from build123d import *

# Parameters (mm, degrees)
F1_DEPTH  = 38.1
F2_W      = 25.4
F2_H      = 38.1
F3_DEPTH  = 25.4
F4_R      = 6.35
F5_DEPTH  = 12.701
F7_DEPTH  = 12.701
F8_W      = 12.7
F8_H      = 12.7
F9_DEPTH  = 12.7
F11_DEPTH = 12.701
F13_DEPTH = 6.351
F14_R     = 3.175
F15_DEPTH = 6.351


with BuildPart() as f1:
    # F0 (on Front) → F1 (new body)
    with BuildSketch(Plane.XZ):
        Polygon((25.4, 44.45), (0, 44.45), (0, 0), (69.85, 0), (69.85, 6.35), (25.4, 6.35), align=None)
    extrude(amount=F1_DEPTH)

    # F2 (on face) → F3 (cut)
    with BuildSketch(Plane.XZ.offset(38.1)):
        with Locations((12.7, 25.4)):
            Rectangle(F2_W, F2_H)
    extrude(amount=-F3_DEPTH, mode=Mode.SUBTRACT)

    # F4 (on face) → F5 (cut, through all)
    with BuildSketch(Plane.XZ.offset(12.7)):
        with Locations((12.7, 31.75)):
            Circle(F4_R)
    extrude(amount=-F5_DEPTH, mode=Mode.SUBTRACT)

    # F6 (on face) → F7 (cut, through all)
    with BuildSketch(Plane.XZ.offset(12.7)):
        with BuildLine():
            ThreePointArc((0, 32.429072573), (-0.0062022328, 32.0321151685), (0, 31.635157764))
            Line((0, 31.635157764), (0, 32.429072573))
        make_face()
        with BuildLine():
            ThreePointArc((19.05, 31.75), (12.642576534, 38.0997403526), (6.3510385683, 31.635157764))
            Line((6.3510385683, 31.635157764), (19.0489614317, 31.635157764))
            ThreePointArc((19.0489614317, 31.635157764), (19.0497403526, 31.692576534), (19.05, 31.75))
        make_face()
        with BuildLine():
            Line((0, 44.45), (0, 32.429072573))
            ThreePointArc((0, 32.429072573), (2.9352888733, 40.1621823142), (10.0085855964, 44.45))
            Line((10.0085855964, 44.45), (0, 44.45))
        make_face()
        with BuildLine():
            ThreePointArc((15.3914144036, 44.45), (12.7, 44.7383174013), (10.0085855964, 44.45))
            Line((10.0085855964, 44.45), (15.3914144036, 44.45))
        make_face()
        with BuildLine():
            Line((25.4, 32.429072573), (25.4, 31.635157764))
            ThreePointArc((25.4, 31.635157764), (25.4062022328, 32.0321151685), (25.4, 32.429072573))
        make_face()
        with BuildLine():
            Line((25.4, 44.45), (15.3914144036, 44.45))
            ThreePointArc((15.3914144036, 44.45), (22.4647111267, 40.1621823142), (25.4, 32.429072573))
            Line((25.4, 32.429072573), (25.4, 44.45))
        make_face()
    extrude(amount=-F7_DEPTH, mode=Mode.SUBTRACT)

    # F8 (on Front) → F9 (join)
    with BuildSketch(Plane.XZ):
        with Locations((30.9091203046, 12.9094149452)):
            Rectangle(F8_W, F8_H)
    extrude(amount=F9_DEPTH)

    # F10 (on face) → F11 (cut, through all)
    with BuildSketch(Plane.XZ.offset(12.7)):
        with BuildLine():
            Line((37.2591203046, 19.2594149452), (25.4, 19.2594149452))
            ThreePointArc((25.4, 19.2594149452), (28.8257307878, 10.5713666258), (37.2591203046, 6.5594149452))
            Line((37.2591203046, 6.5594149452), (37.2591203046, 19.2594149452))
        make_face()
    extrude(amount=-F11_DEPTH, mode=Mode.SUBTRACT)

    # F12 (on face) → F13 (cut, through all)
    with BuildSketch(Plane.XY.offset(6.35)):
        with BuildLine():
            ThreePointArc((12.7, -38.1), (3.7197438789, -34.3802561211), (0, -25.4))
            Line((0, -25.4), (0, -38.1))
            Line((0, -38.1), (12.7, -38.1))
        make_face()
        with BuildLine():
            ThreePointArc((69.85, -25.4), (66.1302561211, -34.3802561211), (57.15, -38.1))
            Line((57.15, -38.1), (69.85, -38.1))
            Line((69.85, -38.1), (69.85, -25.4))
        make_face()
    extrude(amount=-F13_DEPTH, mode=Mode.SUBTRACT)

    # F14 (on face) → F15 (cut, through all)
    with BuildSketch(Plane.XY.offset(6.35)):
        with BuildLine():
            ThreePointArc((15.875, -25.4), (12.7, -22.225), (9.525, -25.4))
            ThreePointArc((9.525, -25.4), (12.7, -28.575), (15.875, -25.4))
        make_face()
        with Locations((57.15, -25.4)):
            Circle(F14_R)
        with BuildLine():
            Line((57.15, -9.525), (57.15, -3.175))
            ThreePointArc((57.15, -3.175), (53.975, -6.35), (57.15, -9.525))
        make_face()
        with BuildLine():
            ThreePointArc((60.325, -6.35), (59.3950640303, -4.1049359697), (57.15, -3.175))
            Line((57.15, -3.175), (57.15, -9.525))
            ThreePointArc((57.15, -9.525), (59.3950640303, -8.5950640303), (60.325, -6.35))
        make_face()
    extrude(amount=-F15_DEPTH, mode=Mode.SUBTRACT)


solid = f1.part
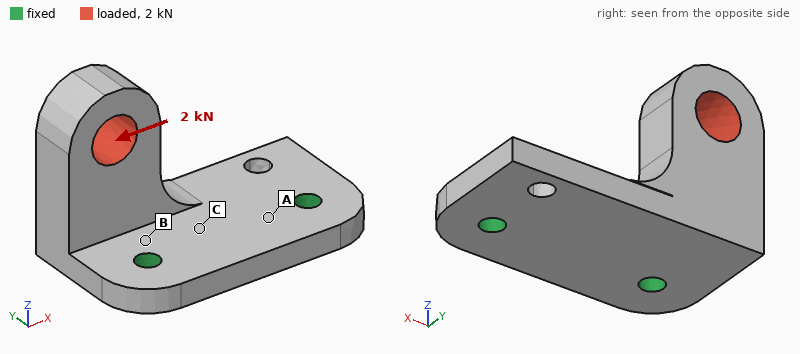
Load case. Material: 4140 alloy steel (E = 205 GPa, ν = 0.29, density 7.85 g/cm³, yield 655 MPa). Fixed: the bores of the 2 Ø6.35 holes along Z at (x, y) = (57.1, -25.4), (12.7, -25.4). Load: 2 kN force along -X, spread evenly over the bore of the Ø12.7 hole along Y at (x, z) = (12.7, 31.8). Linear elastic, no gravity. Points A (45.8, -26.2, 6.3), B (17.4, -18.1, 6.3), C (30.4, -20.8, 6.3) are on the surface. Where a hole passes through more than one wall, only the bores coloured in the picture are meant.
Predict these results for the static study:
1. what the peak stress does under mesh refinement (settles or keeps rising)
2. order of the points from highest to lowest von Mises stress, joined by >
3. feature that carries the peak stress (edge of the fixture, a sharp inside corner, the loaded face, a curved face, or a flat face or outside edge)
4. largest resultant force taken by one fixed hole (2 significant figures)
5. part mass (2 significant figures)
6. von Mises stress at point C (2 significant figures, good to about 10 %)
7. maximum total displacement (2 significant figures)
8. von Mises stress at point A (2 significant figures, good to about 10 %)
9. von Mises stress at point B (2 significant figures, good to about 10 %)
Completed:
keeps rising
B > C > A
a sharp inside corner
1.6 kN
210 g
47 MPa
100 µm
24 MPa
100 MPa
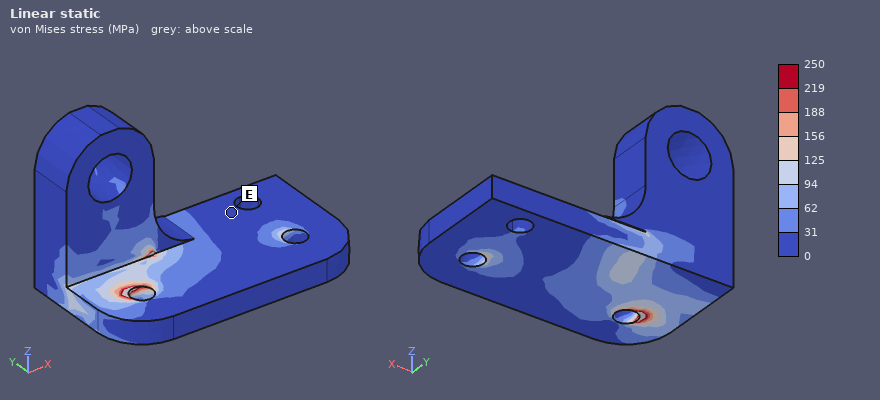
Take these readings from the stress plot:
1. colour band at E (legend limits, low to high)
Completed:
0 to 31 MPa
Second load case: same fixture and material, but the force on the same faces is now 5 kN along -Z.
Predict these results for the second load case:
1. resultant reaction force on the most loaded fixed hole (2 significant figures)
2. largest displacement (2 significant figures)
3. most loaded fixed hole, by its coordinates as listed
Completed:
4.8 kN
0.23 mm
(12.7, -25.4)
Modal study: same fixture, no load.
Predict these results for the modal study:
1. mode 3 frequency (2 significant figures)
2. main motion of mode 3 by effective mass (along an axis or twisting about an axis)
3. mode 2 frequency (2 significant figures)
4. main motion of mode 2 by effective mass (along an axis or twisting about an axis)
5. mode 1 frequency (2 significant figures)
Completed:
7900 Hz
along Z
3600 Hz
along X
2200 Hz
